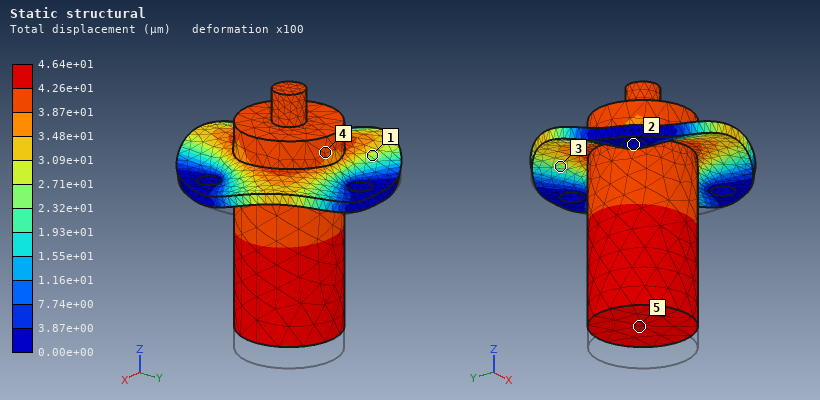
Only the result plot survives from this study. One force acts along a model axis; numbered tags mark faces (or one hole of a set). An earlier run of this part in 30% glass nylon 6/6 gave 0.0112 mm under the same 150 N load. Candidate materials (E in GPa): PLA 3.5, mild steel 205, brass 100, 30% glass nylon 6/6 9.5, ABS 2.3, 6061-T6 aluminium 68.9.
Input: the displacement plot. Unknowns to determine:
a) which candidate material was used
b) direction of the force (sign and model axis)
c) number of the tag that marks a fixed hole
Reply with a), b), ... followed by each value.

a) ABS
b) +Z
c) 2
